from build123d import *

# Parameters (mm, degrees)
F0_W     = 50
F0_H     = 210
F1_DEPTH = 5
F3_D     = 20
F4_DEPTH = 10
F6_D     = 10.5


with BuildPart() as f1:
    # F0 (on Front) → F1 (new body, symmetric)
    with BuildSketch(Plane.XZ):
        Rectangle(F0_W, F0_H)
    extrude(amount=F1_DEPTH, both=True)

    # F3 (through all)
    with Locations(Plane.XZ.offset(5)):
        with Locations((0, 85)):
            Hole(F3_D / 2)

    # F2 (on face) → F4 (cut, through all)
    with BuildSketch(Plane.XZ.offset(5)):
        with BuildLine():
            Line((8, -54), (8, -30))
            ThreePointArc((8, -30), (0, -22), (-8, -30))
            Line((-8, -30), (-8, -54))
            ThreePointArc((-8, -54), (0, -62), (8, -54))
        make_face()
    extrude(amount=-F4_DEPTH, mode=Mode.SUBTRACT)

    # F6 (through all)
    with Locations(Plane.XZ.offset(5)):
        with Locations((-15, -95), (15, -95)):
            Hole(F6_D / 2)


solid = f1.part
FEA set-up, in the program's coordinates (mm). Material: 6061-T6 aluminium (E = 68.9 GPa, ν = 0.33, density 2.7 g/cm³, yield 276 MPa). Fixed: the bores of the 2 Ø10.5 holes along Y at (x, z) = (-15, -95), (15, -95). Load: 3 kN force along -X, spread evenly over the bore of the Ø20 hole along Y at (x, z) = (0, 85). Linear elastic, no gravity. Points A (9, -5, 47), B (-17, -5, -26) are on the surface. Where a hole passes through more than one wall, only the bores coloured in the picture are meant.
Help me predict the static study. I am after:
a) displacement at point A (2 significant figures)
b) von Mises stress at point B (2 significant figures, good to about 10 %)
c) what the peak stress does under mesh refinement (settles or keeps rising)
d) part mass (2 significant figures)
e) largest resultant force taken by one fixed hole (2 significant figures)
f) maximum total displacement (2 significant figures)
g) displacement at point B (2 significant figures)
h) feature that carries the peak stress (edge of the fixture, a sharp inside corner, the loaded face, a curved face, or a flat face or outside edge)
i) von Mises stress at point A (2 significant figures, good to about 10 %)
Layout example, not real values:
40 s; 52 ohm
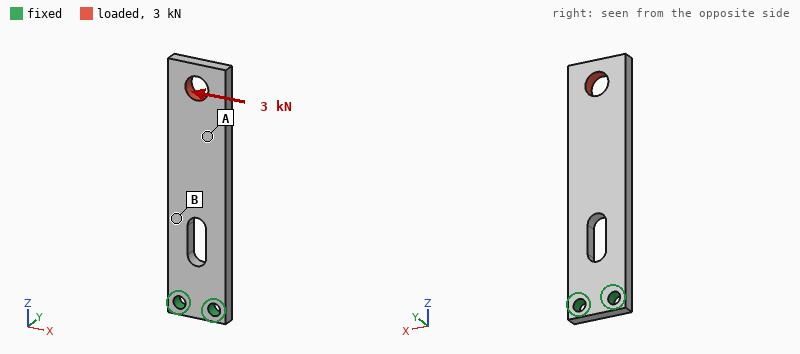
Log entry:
0.64 mm; 54 MPa; keeps rising; 250 g; 15 kN; 1.1 mm; 0.23 mm; edge of the fixture; 17 MPa
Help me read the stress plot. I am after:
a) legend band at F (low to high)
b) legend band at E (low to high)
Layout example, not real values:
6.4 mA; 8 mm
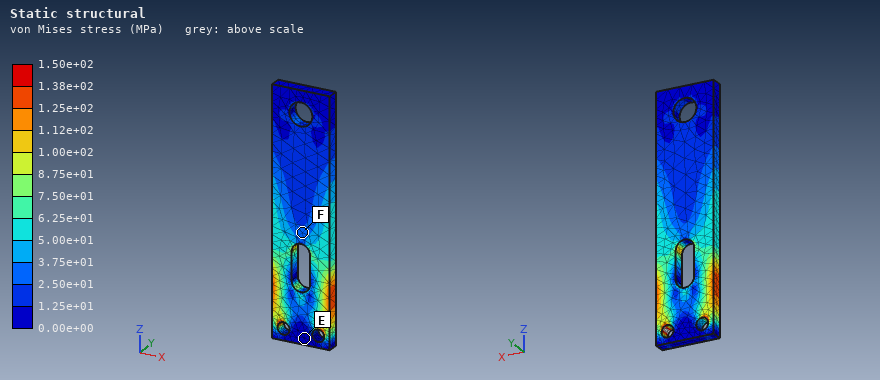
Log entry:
2.50e+01 to 3.75e+01 MPa; 0.00e+00 to 1.25e+01 MPa
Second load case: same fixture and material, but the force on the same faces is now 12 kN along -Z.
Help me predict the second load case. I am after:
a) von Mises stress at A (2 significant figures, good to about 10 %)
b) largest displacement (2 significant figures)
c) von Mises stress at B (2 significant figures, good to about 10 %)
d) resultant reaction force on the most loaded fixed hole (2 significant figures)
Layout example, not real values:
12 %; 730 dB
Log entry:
23 MPa; 89 µm; 33 MPa; 6.0 kN
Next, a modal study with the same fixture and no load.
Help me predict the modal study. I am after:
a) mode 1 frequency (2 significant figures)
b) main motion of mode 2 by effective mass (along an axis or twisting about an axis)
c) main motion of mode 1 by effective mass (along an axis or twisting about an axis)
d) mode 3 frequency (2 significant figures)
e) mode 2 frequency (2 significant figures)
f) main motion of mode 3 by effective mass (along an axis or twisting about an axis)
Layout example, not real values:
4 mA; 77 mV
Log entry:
200 Hz; along X; along Y; 1300 Hz; 980 Hz; along Y
